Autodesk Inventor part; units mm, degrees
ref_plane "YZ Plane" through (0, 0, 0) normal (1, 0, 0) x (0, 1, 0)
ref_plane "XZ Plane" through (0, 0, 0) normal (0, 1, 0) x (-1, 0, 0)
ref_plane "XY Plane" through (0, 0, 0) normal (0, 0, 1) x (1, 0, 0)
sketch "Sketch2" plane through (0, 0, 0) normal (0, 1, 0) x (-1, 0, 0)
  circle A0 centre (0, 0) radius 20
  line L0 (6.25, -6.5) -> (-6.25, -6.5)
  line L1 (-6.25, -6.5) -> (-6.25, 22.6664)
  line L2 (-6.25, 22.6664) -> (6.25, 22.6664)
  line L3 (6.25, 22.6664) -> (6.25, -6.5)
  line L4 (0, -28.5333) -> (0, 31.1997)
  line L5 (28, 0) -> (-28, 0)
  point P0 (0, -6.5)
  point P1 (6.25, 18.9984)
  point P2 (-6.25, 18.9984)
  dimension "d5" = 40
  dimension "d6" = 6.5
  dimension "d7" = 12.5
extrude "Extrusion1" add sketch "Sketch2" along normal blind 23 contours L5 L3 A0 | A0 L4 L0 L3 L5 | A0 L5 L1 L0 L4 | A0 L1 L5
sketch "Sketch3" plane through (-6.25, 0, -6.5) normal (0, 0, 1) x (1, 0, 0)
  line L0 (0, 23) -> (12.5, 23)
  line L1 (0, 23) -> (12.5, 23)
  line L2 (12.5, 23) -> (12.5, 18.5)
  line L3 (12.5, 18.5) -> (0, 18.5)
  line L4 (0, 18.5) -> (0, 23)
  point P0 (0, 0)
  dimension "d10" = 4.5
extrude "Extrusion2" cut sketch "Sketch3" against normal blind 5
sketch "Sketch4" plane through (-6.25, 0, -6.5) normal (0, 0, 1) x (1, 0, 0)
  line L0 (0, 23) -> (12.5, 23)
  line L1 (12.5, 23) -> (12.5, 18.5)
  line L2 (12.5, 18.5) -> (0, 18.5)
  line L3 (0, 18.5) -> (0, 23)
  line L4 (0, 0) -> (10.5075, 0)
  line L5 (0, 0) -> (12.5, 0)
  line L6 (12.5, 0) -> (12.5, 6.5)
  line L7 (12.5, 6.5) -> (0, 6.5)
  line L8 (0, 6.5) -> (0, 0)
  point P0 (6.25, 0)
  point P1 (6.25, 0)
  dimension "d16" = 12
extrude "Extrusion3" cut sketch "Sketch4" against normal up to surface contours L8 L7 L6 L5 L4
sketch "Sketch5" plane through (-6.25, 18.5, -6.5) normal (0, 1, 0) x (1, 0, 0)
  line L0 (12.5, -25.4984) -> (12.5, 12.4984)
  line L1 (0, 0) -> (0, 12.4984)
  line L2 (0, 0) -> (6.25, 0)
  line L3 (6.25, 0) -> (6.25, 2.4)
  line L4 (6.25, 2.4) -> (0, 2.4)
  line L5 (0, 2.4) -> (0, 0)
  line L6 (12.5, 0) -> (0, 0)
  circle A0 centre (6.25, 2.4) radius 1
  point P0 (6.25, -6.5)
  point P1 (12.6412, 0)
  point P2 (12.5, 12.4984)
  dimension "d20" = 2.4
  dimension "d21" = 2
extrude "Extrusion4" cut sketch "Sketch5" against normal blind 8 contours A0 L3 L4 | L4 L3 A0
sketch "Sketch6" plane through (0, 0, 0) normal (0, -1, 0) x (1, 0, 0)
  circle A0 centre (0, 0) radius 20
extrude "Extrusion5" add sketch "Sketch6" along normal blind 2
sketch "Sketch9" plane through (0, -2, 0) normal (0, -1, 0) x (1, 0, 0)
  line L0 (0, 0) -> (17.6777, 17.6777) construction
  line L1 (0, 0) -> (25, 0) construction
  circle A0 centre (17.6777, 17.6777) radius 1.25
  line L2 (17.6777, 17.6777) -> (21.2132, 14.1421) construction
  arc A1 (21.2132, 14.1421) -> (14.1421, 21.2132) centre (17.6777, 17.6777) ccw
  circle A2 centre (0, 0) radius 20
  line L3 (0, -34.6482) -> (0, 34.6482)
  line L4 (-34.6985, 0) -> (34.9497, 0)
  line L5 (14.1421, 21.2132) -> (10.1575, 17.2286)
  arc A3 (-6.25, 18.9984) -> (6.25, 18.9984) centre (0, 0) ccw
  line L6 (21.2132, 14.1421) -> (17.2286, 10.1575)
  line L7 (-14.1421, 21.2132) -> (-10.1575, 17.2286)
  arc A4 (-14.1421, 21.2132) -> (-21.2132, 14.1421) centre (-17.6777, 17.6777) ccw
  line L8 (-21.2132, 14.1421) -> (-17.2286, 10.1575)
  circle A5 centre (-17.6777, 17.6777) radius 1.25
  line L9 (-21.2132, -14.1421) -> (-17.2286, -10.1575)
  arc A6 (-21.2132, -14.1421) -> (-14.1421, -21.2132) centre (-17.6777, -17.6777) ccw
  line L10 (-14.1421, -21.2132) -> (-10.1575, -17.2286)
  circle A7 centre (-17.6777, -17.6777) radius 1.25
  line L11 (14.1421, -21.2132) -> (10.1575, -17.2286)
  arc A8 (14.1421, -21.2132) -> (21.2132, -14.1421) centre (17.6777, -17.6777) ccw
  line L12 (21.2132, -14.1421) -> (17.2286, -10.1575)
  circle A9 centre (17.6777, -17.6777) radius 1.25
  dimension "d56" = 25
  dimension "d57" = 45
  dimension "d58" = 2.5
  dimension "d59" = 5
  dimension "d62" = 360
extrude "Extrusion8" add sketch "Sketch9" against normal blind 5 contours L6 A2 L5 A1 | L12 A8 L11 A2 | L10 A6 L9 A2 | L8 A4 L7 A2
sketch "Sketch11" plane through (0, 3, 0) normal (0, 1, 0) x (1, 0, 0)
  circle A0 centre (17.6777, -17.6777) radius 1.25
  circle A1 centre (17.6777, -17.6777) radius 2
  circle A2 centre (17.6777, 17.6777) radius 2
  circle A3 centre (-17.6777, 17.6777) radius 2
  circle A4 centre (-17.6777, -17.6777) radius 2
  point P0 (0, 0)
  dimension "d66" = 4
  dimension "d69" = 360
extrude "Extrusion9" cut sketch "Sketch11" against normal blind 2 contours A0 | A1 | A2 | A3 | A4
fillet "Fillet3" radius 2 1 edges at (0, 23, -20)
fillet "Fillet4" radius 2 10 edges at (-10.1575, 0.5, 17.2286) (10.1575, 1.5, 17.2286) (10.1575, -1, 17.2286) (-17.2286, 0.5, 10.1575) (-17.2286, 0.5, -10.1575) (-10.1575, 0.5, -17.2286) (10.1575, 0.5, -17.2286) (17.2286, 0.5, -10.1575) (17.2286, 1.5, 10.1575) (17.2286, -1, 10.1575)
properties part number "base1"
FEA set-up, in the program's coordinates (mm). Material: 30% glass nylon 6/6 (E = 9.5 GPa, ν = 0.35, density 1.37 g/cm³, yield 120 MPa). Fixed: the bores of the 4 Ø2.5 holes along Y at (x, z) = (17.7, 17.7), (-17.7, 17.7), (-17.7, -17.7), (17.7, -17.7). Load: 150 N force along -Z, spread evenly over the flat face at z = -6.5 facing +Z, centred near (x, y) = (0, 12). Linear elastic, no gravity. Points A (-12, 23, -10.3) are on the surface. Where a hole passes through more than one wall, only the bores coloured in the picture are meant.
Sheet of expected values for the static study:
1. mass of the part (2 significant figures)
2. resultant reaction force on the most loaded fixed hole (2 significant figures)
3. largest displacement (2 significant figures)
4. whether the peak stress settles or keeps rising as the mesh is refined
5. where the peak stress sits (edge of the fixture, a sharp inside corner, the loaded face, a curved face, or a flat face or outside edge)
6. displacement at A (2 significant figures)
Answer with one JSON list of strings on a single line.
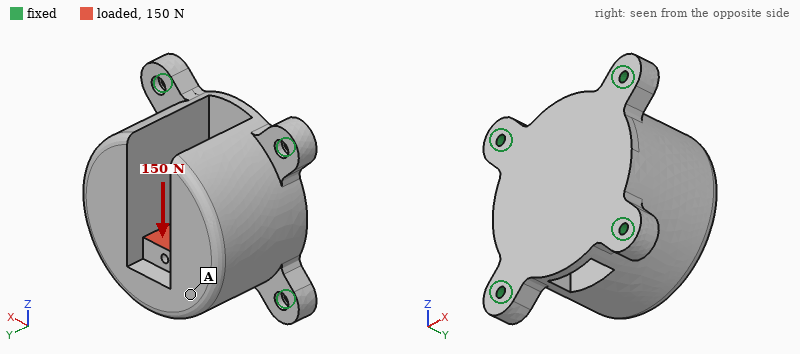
["33 g", "52 N", "6.9 µm", "keeps rising", "edge of the fixture", "5.5 µm"]
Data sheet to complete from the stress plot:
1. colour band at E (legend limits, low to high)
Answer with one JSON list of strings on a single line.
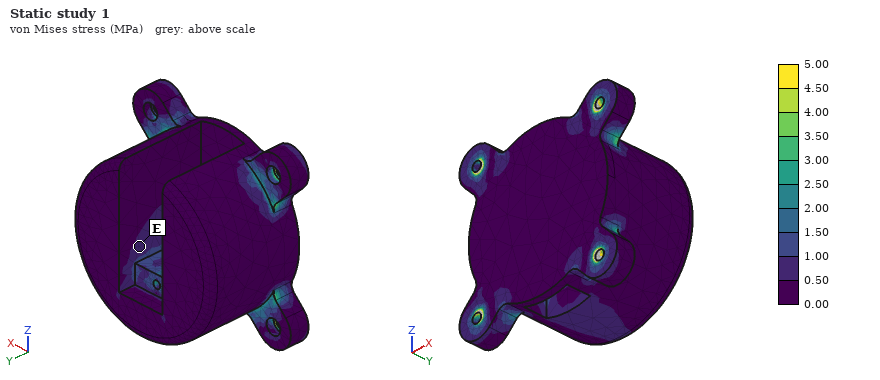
["0.50 to 1.00 MPa"]
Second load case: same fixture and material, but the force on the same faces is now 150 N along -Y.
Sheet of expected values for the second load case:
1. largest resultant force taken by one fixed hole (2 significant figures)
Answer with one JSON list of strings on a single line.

["63 N"]
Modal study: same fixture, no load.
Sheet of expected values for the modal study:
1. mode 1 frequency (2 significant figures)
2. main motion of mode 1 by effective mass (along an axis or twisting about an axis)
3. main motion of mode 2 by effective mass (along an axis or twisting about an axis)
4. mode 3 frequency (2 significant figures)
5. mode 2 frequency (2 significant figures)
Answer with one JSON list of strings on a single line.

["4300 Hz", "along X", "along Y", "5200 Hz", "5000 Hz"]
